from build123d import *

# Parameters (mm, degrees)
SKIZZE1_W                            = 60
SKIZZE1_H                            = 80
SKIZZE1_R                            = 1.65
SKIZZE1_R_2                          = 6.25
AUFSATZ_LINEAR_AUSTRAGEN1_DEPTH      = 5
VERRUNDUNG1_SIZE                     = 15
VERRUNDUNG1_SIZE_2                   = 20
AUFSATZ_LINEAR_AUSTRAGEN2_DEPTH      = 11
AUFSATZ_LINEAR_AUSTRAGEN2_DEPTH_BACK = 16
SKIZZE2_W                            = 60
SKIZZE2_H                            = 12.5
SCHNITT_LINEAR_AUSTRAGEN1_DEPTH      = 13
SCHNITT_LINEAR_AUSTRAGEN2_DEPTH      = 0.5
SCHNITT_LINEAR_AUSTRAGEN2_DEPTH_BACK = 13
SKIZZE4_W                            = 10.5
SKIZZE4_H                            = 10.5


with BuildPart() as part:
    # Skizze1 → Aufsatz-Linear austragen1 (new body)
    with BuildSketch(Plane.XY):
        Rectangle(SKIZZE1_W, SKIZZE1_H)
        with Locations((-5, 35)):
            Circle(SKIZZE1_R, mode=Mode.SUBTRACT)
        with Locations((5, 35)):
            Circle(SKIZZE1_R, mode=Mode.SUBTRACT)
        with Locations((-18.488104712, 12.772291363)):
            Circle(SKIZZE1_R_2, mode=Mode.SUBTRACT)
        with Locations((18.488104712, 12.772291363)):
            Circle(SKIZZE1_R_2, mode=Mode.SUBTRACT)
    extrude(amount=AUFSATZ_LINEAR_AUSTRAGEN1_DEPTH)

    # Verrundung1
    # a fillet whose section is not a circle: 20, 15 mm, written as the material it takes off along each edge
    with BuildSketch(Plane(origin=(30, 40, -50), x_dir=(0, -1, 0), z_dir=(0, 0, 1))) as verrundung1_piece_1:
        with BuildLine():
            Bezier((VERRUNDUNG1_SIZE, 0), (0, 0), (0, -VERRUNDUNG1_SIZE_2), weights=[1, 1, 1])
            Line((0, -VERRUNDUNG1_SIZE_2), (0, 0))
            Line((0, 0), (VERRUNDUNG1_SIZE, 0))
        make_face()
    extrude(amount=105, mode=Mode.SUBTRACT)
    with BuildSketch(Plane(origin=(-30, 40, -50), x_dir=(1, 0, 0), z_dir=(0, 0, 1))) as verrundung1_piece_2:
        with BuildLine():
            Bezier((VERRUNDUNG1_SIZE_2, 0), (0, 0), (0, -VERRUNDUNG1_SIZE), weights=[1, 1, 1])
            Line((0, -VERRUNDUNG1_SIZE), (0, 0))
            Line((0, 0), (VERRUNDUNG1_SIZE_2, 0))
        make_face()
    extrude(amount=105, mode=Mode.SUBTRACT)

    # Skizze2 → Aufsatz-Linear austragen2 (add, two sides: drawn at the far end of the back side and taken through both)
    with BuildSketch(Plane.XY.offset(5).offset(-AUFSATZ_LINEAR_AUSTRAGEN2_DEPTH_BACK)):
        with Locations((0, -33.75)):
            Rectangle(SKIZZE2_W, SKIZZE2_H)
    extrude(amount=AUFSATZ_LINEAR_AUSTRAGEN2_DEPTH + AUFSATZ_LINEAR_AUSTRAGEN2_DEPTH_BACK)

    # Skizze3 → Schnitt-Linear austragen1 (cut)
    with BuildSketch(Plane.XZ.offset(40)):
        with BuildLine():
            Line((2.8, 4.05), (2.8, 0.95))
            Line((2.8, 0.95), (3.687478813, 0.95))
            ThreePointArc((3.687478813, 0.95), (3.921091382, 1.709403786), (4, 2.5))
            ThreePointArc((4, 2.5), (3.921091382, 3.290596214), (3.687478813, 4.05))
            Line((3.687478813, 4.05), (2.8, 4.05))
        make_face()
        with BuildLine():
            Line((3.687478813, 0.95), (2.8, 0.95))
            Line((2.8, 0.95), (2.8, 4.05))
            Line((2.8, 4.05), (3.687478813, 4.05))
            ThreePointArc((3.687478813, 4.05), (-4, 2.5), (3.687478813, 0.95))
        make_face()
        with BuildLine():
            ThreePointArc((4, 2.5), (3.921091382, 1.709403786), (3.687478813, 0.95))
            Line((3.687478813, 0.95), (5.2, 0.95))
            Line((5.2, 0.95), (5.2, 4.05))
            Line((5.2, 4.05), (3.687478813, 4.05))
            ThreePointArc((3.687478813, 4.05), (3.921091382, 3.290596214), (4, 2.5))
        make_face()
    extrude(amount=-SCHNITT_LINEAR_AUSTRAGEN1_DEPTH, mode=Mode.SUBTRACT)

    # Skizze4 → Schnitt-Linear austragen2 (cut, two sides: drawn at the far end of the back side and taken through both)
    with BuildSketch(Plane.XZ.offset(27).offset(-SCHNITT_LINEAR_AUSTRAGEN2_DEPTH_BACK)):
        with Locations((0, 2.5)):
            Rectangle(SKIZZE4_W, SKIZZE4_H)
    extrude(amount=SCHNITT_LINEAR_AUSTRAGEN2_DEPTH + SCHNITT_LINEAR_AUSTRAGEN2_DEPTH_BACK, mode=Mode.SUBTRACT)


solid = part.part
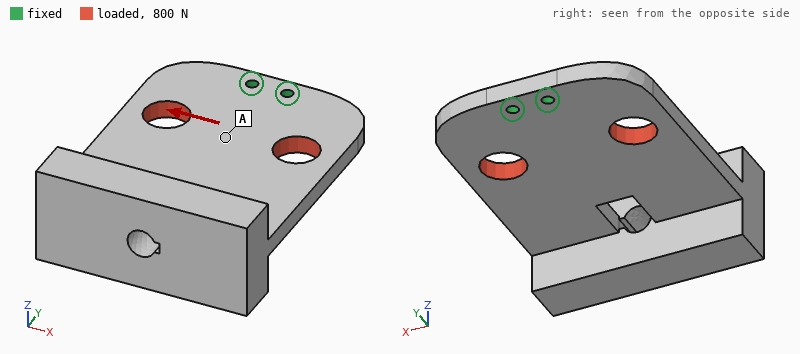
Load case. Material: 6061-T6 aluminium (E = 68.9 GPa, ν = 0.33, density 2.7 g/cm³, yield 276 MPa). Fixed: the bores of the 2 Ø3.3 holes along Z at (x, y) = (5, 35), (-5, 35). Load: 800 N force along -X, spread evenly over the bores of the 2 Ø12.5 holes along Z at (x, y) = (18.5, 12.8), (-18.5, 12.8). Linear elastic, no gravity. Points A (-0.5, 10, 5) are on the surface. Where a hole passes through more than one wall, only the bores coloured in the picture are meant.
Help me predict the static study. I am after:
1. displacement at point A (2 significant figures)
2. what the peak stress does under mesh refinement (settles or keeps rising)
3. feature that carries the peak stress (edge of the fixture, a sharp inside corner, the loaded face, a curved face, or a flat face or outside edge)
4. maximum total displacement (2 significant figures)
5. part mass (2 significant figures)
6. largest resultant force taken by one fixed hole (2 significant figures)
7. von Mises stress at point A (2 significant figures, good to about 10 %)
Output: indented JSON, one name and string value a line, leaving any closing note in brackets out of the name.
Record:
{
  "displacement at point A": "20 µm",
  "what the peak stress does under mesh refinement": "keeps rising",
  "feature that carries the peak stress": "edge of the fixture",
  "maximum total displacement": "60 µm",
  "part mass": "100 g",
  "largest resultant force taken by one fixed hole": "1.4 kN",
  "von Mises stress at point A": "5.9 MPa"
}
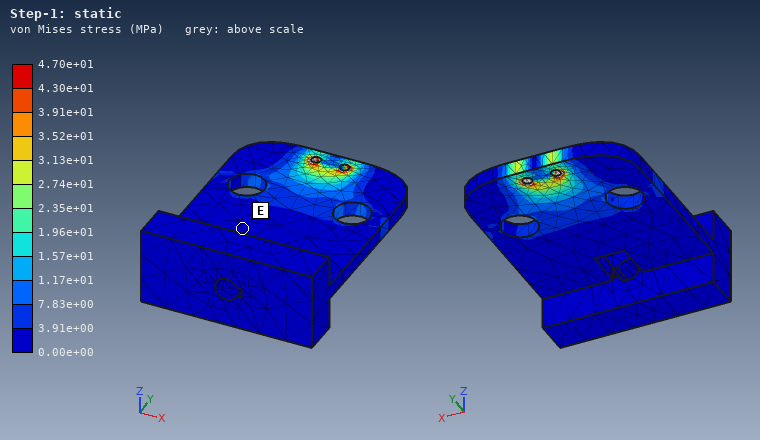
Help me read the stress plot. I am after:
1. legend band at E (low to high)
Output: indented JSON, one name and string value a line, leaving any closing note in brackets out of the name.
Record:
{
  "legend band at E": "0.00e+00 to 3.91e+00 MPa"
}
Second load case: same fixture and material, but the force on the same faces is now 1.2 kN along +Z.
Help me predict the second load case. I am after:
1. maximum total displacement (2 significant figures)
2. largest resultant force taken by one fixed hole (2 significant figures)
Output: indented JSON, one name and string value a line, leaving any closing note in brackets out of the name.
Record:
{
  "maximum total displacement": "0.76 mm",
  "largest resultant force taken by one fixed hole": "600 N"
}
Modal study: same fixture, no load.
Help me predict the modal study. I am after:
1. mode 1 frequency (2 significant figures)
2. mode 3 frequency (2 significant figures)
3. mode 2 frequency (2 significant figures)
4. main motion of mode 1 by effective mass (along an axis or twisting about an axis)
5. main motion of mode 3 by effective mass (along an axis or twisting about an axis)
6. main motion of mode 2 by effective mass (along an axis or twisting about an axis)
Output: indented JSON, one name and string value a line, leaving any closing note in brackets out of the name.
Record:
{
  "mode 1 frequency": "330 Hz",
  "mode 3 frequency": "1300 Hz",
  "mode 2 frequency": "980 Hz",
  "main motion of mode 1 by effective mass": "along Z",
  "main motion of mode 3 by effective mass": "along X",
  "main motion of mode 2 by effective mass": "twisting about Y"
}
